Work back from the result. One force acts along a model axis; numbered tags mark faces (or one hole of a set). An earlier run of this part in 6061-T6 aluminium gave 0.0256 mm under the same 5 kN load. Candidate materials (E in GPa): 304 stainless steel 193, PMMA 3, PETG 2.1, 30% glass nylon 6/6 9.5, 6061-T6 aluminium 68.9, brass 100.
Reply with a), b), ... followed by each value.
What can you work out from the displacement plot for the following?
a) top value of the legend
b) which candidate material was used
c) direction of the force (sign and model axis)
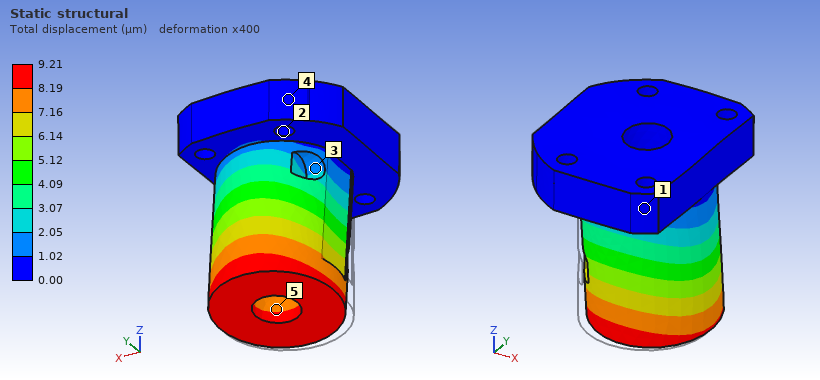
a) 9.21 µm
b) 304 stainless steel
c) +Y
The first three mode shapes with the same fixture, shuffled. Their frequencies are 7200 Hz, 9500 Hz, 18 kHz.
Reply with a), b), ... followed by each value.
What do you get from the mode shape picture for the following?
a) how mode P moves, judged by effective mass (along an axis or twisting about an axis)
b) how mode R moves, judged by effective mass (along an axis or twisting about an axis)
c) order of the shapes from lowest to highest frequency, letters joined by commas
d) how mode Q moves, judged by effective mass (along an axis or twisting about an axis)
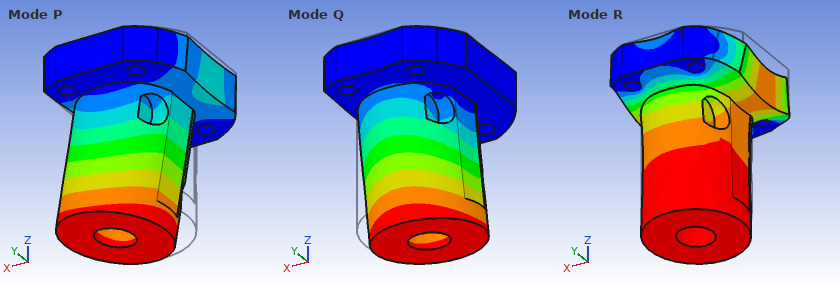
a) along X
b) along Z
c) P, Q, R
d) along Y
